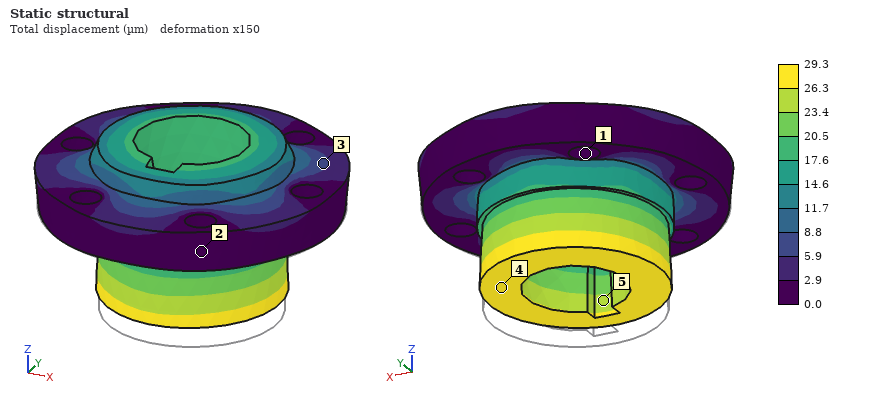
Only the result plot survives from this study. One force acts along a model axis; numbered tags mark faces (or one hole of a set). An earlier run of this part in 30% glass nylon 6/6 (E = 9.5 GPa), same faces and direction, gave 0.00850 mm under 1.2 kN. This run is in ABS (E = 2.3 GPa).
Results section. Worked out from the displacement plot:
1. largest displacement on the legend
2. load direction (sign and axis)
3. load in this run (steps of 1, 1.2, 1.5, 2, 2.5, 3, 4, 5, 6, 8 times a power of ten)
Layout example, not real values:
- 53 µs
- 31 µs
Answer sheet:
- 29.3 µm
- +Z
- 1 kN
